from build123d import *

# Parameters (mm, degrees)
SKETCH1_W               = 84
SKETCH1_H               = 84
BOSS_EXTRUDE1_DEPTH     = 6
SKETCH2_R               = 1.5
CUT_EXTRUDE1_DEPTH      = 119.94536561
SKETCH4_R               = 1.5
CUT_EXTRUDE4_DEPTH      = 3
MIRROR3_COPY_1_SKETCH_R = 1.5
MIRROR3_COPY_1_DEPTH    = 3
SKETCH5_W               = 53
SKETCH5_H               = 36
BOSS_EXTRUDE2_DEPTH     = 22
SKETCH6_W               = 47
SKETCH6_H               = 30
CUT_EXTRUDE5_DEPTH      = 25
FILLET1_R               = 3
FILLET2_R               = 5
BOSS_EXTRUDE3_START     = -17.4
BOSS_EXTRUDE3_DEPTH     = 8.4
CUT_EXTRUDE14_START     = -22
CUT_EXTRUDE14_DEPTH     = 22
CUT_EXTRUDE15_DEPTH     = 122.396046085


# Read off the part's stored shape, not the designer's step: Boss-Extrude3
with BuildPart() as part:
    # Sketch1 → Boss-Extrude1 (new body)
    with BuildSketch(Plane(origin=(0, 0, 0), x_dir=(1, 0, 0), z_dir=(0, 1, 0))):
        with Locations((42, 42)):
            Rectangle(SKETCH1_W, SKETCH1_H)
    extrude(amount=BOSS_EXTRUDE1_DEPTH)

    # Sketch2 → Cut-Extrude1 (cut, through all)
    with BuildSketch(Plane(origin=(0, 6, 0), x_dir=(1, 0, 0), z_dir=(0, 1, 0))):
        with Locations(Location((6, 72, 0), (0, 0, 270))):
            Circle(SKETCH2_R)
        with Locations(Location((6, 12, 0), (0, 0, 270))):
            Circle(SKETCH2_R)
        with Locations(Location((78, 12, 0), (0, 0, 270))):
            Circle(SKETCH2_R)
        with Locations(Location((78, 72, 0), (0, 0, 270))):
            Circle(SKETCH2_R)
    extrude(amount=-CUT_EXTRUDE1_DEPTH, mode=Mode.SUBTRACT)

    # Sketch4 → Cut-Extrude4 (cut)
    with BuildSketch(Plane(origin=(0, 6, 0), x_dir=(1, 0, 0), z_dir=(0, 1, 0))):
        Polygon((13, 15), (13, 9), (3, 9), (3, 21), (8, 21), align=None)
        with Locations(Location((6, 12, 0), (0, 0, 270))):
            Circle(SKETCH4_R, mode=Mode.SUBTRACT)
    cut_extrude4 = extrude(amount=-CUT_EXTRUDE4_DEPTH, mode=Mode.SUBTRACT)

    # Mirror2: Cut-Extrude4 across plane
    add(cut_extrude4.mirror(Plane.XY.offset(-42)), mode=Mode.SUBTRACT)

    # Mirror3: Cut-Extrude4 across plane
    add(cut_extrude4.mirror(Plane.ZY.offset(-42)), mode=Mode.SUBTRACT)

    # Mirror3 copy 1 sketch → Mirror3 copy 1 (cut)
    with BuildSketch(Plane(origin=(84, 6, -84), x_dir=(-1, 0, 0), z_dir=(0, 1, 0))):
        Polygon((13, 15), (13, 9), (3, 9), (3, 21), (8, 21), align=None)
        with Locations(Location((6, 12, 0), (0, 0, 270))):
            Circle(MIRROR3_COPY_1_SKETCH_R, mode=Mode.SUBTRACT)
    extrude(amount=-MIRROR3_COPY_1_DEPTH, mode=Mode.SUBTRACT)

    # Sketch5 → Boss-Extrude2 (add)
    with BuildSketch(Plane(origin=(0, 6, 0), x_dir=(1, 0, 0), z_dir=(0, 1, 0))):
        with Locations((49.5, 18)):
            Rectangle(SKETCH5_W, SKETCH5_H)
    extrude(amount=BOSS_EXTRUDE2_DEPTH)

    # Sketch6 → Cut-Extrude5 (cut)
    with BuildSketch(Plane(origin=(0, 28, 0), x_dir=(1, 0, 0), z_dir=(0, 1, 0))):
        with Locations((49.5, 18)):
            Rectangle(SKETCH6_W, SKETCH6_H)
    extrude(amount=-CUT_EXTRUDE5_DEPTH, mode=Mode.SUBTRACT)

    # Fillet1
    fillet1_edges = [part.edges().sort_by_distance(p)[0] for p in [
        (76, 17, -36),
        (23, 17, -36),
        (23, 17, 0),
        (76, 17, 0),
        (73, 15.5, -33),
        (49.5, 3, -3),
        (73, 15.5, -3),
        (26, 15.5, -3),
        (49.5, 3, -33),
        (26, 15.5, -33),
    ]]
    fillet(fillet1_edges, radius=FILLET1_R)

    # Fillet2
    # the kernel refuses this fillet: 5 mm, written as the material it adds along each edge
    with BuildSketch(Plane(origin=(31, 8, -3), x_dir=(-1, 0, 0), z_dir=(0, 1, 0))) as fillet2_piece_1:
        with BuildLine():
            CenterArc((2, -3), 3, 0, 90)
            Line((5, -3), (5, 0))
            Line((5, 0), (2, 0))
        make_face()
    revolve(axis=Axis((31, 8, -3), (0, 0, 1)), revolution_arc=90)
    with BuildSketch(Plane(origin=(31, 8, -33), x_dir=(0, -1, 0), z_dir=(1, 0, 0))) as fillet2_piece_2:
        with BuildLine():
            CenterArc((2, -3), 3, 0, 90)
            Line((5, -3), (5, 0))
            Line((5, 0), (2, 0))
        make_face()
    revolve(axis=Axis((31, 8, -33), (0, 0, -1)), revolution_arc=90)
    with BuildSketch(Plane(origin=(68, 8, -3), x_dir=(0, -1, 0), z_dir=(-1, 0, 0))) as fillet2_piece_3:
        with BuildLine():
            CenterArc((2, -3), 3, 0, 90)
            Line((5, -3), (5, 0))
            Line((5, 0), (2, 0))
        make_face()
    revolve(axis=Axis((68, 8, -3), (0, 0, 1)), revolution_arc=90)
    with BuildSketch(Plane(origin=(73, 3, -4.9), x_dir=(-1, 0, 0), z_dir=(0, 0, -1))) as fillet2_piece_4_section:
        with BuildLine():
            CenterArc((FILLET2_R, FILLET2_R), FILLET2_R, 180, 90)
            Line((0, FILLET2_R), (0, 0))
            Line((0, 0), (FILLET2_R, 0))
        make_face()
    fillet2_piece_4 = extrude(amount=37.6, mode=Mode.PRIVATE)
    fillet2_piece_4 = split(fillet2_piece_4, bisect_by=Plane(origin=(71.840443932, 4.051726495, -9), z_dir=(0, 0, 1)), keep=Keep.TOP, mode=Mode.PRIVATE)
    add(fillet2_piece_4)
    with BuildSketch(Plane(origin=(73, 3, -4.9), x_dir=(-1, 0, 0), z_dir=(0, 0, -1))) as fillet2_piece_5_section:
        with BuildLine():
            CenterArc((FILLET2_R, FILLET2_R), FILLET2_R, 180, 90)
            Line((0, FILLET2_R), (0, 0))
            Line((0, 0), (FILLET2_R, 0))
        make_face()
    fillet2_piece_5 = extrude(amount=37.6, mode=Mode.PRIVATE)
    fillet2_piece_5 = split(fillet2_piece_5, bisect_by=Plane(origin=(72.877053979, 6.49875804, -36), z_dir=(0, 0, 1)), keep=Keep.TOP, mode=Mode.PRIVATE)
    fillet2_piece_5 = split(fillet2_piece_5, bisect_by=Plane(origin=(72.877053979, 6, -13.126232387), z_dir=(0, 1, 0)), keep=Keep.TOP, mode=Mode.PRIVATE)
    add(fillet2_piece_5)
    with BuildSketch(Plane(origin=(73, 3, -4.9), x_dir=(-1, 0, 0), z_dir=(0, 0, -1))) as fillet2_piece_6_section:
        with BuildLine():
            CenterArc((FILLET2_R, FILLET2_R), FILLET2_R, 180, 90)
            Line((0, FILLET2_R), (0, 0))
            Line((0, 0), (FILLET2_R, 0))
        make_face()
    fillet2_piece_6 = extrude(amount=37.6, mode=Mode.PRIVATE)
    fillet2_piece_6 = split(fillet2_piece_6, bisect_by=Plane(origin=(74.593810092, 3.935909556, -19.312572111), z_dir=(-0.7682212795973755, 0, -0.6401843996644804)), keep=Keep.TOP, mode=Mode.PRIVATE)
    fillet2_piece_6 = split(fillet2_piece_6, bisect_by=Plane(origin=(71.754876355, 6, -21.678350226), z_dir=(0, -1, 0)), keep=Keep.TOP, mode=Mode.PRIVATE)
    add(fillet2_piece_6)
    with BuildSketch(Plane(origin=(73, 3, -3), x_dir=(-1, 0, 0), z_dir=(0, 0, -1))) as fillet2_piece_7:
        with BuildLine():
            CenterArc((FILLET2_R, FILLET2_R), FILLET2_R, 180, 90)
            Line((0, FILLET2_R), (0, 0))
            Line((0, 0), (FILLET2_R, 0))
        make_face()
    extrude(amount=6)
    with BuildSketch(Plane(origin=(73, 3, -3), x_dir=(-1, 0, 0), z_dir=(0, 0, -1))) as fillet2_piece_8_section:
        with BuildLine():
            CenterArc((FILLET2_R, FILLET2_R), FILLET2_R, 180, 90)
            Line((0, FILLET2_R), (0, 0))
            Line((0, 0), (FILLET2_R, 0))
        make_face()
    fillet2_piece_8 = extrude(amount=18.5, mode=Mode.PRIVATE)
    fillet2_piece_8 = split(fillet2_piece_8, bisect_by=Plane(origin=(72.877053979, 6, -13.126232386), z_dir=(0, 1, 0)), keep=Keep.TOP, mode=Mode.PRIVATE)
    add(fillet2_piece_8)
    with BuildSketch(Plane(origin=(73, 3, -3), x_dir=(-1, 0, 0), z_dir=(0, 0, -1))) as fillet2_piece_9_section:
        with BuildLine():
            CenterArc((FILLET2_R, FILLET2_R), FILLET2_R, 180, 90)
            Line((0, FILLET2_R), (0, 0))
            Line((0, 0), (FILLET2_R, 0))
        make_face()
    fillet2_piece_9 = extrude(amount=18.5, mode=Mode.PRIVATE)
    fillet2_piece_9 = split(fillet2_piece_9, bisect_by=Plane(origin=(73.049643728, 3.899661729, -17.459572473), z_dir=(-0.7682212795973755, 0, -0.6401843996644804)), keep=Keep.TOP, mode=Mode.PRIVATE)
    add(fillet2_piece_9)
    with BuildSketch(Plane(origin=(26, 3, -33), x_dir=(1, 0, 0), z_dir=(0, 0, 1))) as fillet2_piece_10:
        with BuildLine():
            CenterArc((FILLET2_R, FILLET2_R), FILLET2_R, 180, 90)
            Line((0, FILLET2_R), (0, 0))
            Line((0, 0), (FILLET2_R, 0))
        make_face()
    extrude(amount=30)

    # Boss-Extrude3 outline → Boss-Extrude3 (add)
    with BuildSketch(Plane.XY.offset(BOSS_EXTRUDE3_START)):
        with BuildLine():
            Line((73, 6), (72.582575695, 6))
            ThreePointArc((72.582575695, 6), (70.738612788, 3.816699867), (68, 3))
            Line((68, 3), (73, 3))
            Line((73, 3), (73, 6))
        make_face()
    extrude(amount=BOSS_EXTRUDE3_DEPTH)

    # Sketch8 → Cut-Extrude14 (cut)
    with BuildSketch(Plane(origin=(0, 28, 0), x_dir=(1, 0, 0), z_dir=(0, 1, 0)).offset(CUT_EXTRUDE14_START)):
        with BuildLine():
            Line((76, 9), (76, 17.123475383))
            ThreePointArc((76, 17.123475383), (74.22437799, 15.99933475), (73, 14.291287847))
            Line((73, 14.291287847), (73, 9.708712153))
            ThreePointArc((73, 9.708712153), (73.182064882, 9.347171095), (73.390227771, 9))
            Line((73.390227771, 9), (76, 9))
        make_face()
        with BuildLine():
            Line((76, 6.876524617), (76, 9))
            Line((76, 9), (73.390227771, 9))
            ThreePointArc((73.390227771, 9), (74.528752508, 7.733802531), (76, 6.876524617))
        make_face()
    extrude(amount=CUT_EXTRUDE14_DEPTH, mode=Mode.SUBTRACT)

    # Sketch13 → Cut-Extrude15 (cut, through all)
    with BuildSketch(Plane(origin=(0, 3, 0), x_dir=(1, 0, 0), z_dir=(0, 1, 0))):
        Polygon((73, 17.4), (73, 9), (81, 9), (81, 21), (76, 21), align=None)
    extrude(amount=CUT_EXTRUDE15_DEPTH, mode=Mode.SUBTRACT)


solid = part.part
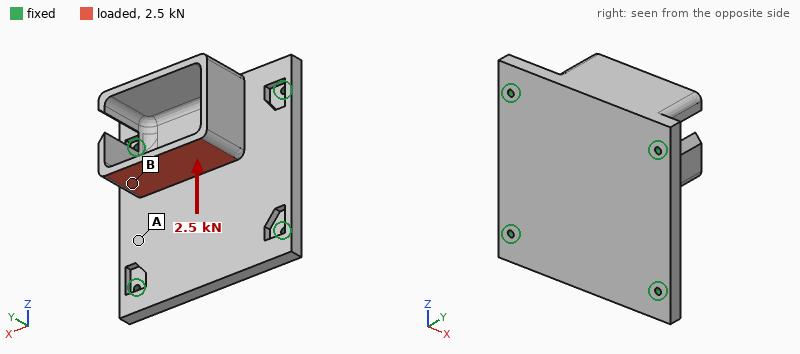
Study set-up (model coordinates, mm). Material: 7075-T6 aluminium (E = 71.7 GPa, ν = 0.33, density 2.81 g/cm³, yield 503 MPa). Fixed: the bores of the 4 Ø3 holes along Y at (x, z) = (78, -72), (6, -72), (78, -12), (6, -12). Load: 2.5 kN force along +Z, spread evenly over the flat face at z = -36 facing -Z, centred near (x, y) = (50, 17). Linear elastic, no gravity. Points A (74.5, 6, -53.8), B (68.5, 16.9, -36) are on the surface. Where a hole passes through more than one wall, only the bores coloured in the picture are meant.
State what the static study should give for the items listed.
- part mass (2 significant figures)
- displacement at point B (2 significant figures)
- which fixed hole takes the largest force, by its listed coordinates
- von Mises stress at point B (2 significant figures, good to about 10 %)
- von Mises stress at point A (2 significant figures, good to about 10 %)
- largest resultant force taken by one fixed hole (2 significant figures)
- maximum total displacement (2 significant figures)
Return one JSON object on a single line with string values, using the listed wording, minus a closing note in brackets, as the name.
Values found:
{"part mass": "130 g", "displacement at point B": "0.071 mm", "which fixed hole takes the largest force, by its listed coordinates": "(78, -72)", "von Mises stress at point B": "71 MPa", "von Mises stress at point A": "20 MPa", "largest resultant force taken by one fixed hole": "1.1 kN", "maximum total displacement": "0.26 mm"}
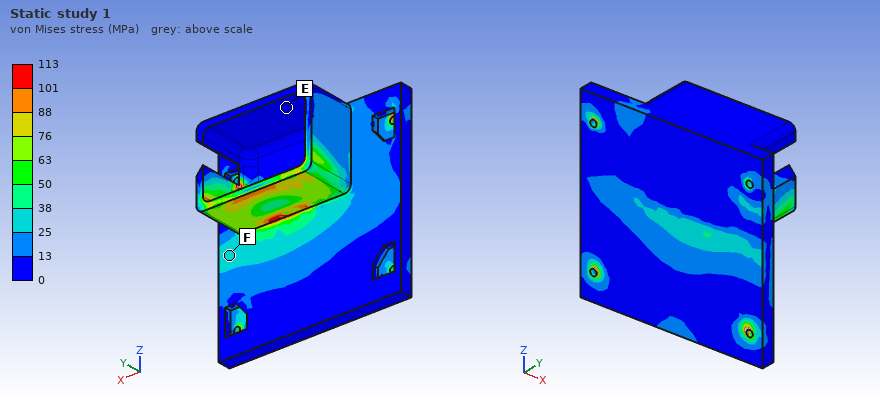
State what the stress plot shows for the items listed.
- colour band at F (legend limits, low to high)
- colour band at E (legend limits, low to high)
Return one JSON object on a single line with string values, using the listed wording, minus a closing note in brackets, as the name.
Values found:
{"colour band at F": "25 to 38 MPa", "colour band at E": "0 to 13 MPa"}
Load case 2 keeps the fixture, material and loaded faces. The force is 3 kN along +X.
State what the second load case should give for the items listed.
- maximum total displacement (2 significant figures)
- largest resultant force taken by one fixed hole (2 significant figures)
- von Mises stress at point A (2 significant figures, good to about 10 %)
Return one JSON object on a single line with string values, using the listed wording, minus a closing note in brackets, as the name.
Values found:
{"maximum total displacement": "69 µm", "largest resultant force taken by one fixed hole": "1.1 kN", "von Mises stress at point A": "17 MPa"}
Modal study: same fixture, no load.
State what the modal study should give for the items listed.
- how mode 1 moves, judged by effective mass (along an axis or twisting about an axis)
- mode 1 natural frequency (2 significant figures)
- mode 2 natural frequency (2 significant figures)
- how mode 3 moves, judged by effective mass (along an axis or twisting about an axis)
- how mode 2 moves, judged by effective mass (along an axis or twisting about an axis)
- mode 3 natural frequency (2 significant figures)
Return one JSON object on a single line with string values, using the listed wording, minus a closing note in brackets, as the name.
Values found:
{"how mode 1 moves, judged by effective mass": "along Y", "mode 1 natural frequency": "3200 Hz", "mode 2 natural frequency": "3800 Hz", "how mode 3 moves, judged by effective mass": "twisting about X", "how mode 2 moves, judged by effective mass": "along Y", "mode 3 natural frequency": "4800 Hz"}
